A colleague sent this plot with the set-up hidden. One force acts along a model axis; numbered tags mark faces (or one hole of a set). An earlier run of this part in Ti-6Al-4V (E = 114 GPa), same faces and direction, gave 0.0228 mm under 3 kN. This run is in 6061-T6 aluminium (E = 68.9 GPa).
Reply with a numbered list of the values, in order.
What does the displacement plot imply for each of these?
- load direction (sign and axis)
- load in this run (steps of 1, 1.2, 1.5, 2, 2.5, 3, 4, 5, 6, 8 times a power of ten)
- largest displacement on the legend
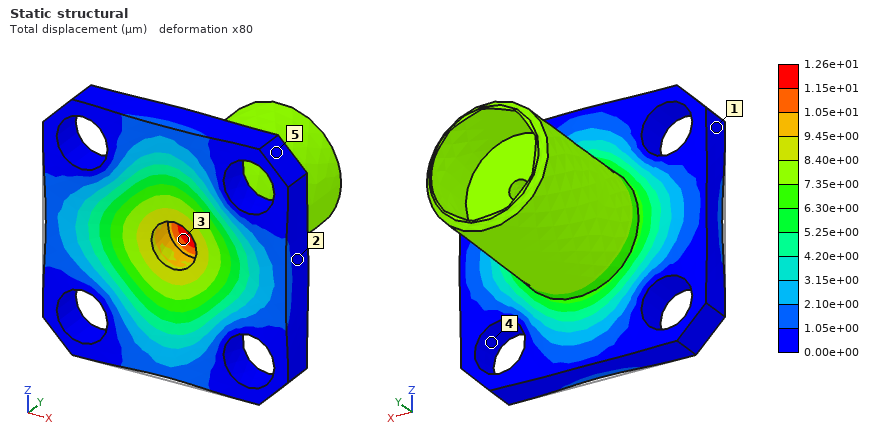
1. +Y
2. 1 kN
3. 1.26e+01 µm
